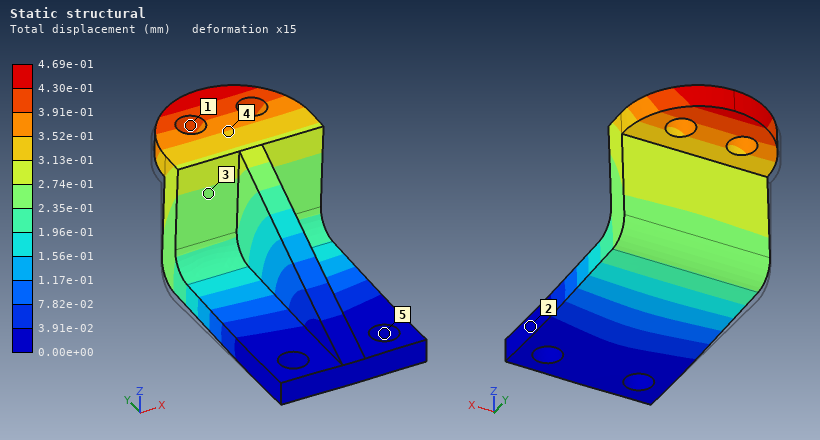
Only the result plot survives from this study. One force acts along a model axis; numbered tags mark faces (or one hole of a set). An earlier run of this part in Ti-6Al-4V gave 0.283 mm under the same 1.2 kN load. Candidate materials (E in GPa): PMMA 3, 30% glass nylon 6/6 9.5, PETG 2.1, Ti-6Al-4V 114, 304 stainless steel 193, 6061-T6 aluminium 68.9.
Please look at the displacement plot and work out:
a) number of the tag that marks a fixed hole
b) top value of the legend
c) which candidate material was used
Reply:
5
4.69e-01 mm
6061-T6 aluminium
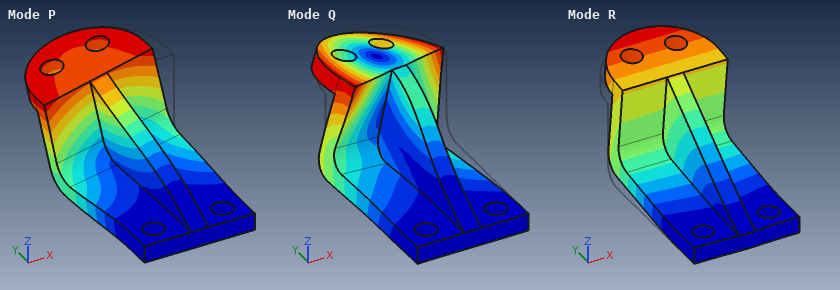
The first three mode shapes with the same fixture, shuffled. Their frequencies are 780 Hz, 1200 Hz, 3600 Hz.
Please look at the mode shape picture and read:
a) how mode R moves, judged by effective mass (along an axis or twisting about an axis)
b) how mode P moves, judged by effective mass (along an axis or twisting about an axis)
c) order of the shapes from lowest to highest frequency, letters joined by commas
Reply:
along Z
along X
R, P, Q
